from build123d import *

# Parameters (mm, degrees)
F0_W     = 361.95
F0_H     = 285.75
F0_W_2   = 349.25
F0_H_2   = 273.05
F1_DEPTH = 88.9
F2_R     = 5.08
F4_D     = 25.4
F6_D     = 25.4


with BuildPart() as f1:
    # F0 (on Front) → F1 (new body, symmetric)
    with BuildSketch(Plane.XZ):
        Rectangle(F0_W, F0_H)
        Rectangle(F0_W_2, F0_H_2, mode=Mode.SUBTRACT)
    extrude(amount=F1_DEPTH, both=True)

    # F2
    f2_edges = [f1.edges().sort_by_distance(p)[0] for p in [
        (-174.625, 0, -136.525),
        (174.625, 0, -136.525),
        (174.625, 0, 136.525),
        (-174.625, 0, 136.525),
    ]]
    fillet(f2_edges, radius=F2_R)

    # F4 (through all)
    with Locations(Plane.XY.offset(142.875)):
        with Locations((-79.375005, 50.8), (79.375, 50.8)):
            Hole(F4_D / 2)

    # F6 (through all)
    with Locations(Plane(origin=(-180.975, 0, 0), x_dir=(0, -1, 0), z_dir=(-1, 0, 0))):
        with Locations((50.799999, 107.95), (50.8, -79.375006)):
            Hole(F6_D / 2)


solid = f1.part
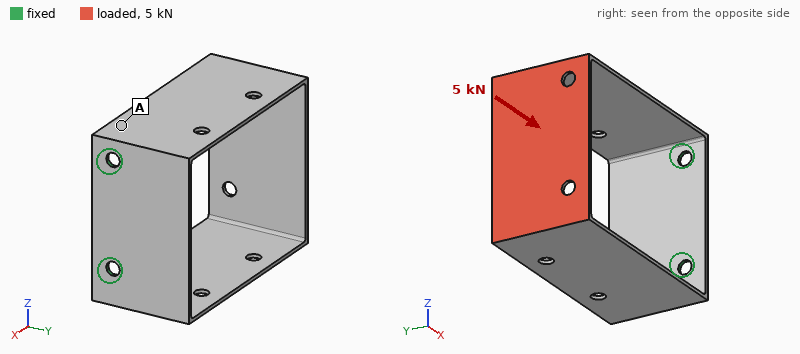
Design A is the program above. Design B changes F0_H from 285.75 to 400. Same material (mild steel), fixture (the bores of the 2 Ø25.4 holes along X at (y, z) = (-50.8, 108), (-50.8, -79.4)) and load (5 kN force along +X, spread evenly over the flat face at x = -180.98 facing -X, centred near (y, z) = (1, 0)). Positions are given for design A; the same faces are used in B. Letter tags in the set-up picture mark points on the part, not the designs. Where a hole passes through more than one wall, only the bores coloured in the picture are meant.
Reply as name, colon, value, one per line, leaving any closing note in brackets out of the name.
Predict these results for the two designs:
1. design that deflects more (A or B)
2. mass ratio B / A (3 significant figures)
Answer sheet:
design that deflects more: A
mass ratio B / A: 6.12
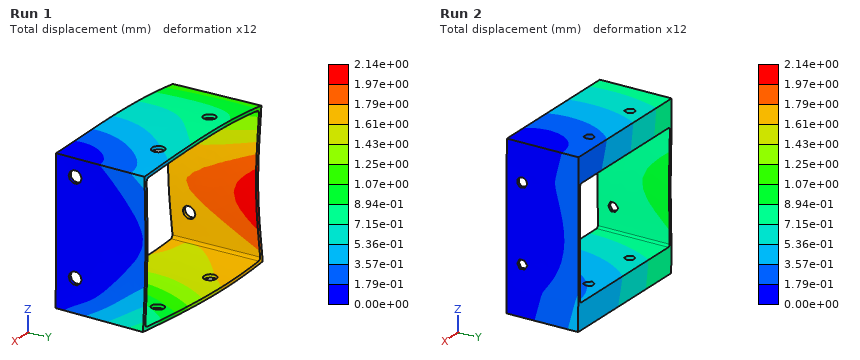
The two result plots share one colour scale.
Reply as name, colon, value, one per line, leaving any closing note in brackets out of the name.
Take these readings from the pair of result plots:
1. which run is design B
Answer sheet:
which run is design B: Run 2
